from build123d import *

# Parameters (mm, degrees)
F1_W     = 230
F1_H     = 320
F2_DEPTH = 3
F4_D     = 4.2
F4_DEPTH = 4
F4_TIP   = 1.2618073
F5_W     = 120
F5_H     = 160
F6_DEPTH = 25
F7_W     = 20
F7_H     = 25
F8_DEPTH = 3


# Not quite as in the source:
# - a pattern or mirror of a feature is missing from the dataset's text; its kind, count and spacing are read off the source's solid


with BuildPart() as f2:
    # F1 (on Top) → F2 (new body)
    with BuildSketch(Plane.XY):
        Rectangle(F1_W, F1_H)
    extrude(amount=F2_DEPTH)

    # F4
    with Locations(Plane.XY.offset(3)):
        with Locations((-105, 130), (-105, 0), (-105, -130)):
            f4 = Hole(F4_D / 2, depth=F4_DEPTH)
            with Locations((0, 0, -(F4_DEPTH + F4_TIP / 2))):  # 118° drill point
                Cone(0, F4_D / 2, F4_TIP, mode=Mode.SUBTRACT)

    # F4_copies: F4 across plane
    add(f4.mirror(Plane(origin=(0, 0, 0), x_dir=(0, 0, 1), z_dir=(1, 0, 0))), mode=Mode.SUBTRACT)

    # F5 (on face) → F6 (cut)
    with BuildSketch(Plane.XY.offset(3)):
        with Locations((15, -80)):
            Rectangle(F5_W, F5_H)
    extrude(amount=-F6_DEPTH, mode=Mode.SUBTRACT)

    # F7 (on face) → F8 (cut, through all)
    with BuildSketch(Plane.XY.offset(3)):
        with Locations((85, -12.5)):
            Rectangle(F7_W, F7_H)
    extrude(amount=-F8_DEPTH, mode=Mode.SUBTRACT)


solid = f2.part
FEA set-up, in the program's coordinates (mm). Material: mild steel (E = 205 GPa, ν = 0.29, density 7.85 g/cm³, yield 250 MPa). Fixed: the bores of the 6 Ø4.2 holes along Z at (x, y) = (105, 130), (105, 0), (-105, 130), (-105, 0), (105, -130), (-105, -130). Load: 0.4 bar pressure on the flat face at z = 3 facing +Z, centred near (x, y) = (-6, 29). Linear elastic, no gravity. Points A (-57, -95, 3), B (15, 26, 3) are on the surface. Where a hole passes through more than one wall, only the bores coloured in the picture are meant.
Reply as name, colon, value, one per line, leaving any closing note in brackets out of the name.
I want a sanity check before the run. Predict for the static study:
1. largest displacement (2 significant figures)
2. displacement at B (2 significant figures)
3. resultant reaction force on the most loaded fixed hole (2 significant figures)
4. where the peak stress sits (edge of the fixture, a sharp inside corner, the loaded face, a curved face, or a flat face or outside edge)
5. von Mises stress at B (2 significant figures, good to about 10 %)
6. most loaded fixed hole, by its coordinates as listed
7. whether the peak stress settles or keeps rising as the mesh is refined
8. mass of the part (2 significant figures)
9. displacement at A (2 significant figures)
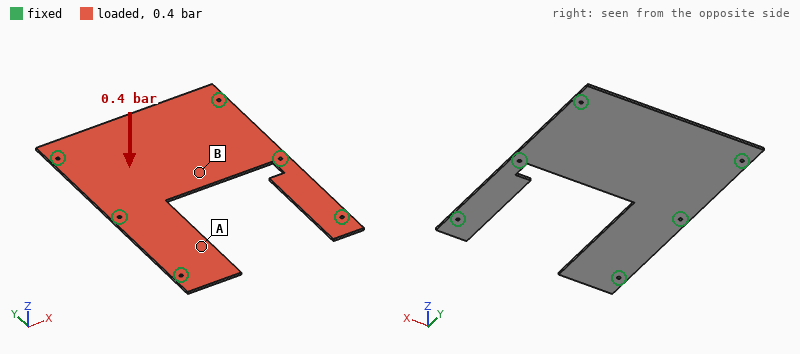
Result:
largest displacement: 0.71 mm
displacement at B: 0.68 mm
resultant reaction force on the most loaded fixed hole: 510 N
where the peak stress sits: edge of the fixture
von Mises stress at B: 57 MPa
most loaded fixed hole, by its coordinates as listed: (-105, 0)
whether the peak stress settles or keeps rising as the mesh is refined: keeps rising
mass of the part: 1.3 kg
displacement at A: 0.32 mm
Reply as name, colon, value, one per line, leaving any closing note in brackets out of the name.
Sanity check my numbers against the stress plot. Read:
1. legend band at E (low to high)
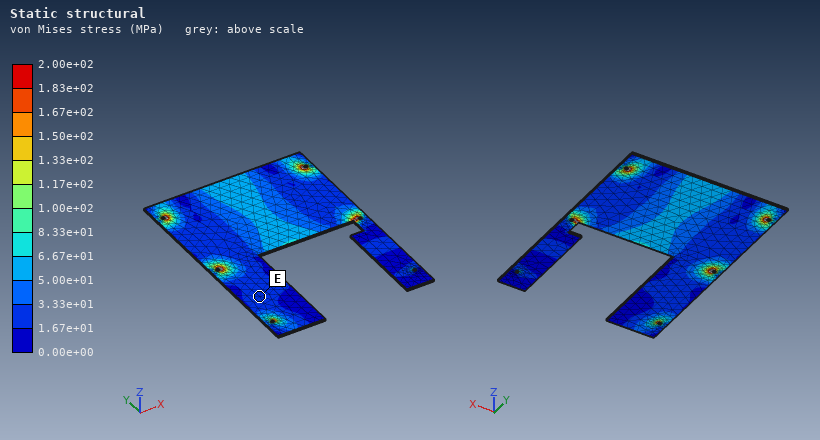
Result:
legend band at E: 1.67e+01 to 3.33e+01 MPa
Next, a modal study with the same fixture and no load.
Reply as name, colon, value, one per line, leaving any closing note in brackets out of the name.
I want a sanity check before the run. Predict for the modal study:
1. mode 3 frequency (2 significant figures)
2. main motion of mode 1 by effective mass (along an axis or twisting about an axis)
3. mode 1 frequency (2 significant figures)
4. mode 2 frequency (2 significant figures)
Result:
mode 3 frequency: 530 Hz
main motion of mode 1 by effective mass: along Z
mode 1 frequency: 290 Hz
mode 2 frequency: 430 Hz
